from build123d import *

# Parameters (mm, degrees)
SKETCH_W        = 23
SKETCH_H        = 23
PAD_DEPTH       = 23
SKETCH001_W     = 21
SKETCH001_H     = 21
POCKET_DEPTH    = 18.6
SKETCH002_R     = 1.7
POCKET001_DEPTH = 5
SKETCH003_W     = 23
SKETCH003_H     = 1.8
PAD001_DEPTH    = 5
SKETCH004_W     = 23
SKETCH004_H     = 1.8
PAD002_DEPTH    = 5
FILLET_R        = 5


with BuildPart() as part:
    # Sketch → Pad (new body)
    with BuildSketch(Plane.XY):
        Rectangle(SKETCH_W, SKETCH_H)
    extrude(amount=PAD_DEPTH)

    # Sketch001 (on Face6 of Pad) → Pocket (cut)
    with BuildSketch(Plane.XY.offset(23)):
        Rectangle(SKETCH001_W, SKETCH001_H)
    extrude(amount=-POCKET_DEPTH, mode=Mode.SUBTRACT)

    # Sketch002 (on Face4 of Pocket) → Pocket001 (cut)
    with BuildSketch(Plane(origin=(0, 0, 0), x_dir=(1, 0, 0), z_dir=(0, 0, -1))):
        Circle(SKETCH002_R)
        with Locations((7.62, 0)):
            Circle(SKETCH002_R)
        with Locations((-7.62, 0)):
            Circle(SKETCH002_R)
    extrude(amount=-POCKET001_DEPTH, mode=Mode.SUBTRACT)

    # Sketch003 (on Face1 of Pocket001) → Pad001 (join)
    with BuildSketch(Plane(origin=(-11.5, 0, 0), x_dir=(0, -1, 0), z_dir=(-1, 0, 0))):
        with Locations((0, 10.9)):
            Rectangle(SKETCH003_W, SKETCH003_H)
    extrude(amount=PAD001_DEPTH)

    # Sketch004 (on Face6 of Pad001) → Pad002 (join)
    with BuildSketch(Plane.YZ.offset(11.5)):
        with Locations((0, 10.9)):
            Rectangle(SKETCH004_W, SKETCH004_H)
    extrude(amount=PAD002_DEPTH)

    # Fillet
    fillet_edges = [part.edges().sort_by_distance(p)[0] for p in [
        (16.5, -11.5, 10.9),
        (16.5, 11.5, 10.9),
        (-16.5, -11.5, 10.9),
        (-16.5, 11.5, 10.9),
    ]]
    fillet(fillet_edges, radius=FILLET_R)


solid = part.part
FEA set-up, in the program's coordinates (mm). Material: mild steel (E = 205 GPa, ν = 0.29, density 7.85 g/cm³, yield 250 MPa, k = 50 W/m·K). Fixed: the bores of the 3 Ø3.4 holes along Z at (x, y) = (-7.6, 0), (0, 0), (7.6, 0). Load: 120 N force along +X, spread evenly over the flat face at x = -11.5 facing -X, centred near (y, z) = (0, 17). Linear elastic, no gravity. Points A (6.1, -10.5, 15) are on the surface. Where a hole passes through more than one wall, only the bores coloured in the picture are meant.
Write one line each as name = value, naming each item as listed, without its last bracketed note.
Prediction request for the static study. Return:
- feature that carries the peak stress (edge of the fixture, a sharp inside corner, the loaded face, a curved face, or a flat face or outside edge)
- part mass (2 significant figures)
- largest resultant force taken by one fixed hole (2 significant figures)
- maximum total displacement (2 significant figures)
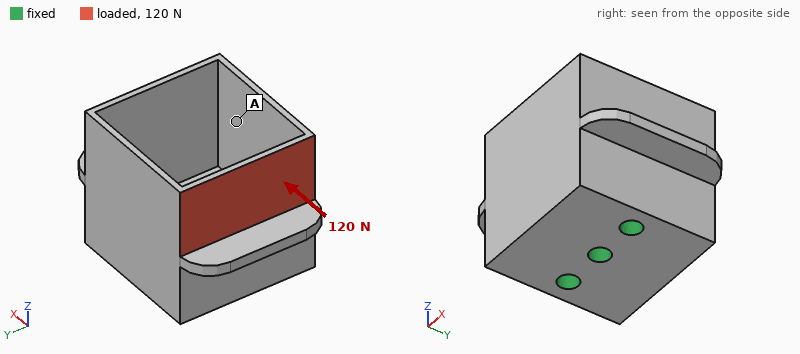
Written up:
feature that carries the peak stress = the loaded face
part mass = 33 g
largest resultant force taken by one fixed hole = 99 N
maximum total displacement = 23 µm
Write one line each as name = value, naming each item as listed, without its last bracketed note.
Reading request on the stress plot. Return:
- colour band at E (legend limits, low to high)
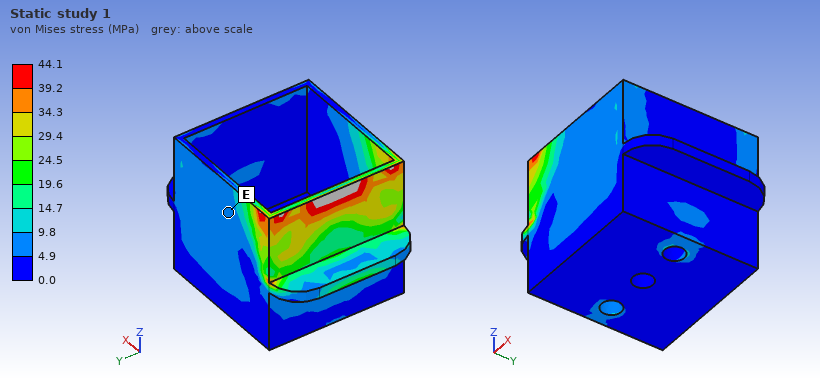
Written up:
colour band at E = 4.9 to 9.8 MPa
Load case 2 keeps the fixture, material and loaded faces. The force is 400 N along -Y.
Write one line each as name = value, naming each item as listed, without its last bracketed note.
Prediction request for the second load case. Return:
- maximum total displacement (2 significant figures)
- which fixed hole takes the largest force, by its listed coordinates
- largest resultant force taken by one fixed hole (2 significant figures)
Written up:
maximum total displacement = 18 µm
which fixed hole takes the largest force, by its listed coordinates = (-7.6, 0)
largest resultant force taken by one fixed hole = 460 N
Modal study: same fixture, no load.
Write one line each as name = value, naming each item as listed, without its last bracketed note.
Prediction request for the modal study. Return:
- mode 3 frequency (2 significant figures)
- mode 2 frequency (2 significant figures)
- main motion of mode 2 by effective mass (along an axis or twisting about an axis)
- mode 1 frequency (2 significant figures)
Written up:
mode 3 frequency = 10 kHz
mode 2 frequency = 8700 Hz
main motion of mode 2 by effective mass = along Y
mode 1 frequency = 8200 Hz
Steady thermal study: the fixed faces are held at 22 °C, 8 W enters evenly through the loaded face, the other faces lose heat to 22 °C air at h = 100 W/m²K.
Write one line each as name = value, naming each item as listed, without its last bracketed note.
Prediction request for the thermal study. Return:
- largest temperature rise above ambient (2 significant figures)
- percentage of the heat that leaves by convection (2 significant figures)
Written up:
largest temperature rise above ambient = 45 K
percentage of the heat that leaves by convection = 49 %
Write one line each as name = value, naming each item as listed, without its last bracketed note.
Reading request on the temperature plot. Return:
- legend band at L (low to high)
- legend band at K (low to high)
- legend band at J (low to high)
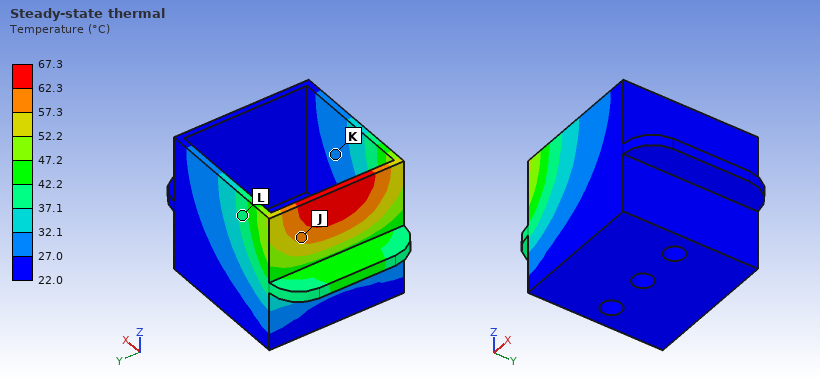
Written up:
legend band at L = 37.1 to 42.2 °C
legend band at K = 27.0 to 32.1 °C
legend band at J = 57.3 to 62.3 °C
